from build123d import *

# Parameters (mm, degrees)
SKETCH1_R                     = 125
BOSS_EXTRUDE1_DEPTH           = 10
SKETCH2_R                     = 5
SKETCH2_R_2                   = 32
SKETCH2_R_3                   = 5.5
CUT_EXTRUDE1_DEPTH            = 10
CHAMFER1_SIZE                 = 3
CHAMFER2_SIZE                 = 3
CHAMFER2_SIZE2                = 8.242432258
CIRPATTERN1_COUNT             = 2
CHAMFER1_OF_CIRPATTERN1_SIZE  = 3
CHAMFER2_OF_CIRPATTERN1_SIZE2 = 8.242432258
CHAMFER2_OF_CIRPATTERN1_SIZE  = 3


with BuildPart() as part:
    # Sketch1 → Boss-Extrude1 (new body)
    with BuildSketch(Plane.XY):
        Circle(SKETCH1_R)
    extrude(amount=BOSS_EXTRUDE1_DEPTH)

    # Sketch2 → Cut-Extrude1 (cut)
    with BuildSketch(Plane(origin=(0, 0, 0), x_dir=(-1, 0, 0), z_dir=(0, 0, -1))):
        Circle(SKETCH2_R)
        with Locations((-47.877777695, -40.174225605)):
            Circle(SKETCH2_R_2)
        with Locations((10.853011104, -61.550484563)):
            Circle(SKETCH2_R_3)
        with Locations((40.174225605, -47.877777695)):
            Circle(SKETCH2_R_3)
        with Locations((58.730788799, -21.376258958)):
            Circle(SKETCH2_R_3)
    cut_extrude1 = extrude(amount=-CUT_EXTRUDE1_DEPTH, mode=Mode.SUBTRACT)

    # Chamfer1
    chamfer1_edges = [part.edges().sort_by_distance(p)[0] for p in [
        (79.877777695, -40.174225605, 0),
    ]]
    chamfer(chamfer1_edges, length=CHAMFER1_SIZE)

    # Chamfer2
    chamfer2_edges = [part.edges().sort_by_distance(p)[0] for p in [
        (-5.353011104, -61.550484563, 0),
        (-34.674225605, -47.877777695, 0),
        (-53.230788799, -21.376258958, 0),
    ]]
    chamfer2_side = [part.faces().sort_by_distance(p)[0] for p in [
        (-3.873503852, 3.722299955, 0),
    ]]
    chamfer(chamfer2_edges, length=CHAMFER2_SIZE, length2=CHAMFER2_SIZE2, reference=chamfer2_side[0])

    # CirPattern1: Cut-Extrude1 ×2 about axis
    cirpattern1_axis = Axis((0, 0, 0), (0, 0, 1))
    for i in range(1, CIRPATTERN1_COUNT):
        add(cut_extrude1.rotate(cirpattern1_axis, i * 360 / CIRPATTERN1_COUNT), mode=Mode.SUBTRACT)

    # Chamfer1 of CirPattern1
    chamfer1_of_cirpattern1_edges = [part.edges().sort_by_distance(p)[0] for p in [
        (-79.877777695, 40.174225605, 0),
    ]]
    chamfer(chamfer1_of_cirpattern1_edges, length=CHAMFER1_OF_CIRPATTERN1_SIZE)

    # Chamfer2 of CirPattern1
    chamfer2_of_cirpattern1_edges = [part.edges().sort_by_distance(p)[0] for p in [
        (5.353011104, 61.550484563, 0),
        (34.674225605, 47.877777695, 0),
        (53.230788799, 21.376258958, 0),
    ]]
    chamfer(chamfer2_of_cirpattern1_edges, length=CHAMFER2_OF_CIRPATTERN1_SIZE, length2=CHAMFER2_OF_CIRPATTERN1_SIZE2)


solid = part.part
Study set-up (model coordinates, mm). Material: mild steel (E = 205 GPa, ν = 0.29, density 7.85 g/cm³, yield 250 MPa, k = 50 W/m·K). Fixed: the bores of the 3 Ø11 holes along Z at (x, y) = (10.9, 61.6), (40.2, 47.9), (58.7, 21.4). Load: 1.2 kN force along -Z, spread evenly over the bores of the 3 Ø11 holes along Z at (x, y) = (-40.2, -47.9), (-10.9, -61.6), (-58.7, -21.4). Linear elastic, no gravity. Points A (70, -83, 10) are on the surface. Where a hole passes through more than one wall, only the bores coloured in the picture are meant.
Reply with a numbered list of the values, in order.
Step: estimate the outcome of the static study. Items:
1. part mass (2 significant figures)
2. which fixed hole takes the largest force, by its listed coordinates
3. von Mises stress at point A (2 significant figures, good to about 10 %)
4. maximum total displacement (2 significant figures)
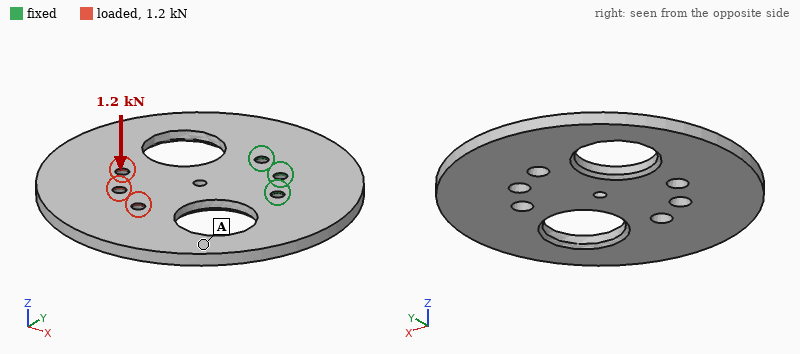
1. 3.3 kg
2. (40.2, 47.9)
3. 23 MPa
4. 0.71 mm
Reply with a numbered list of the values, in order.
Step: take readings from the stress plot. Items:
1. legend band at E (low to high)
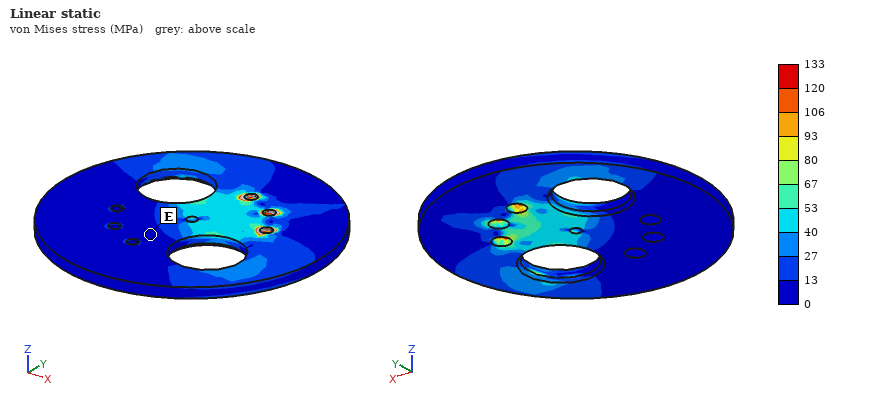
1. 0 to 13 MPa
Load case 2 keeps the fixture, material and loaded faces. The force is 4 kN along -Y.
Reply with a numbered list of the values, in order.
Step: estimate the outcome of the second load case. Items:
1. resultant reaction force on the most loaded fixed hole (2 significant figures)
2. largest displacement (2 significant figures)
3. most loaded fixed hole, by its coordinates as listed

1. 5.5 kN
2. 87 µm
3. (10.9, 61.6)
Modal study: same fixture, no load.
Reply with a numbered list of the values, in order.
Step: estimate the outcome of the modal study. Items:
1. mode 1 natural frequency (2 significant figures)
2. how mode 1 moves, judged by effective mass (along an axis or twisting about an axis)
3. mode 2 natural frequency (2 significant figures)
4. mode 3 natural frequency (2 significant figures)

1. 200 Hz
2. along Z
3. 450 Hz
4. 840 Hz
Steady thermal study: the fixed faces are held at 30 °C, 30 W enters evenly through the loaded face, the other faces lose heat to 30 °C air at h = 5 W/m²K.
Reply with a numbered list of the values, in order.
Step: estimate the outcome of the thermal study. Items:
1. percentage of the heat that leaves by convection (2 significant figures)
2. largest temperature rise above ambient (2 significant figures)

1. 36 %
2. 54 K
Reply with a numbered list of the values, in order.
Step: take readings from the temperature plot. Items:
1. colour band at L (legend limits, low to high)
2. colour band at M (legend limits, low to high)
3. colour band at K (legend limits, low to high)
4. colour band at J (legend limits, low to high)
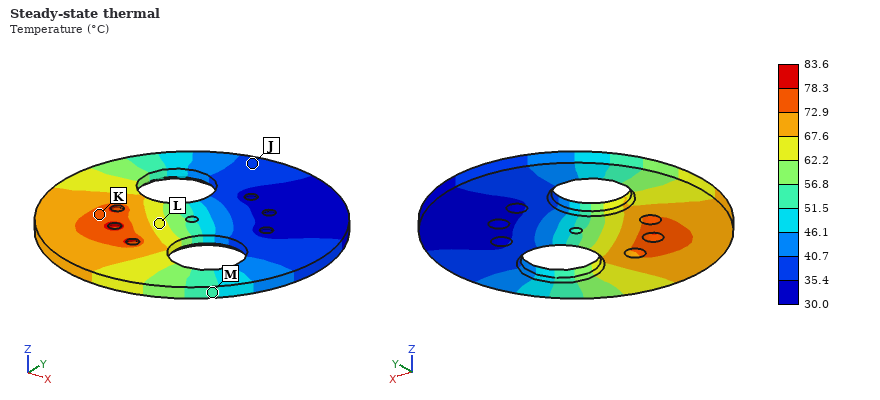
1. 62.2 to 67.6 °C
2. 51.5 to 56.8 °C
3. 72.9 to 78.3 °C
4. 35.4 to 40.7 °C
